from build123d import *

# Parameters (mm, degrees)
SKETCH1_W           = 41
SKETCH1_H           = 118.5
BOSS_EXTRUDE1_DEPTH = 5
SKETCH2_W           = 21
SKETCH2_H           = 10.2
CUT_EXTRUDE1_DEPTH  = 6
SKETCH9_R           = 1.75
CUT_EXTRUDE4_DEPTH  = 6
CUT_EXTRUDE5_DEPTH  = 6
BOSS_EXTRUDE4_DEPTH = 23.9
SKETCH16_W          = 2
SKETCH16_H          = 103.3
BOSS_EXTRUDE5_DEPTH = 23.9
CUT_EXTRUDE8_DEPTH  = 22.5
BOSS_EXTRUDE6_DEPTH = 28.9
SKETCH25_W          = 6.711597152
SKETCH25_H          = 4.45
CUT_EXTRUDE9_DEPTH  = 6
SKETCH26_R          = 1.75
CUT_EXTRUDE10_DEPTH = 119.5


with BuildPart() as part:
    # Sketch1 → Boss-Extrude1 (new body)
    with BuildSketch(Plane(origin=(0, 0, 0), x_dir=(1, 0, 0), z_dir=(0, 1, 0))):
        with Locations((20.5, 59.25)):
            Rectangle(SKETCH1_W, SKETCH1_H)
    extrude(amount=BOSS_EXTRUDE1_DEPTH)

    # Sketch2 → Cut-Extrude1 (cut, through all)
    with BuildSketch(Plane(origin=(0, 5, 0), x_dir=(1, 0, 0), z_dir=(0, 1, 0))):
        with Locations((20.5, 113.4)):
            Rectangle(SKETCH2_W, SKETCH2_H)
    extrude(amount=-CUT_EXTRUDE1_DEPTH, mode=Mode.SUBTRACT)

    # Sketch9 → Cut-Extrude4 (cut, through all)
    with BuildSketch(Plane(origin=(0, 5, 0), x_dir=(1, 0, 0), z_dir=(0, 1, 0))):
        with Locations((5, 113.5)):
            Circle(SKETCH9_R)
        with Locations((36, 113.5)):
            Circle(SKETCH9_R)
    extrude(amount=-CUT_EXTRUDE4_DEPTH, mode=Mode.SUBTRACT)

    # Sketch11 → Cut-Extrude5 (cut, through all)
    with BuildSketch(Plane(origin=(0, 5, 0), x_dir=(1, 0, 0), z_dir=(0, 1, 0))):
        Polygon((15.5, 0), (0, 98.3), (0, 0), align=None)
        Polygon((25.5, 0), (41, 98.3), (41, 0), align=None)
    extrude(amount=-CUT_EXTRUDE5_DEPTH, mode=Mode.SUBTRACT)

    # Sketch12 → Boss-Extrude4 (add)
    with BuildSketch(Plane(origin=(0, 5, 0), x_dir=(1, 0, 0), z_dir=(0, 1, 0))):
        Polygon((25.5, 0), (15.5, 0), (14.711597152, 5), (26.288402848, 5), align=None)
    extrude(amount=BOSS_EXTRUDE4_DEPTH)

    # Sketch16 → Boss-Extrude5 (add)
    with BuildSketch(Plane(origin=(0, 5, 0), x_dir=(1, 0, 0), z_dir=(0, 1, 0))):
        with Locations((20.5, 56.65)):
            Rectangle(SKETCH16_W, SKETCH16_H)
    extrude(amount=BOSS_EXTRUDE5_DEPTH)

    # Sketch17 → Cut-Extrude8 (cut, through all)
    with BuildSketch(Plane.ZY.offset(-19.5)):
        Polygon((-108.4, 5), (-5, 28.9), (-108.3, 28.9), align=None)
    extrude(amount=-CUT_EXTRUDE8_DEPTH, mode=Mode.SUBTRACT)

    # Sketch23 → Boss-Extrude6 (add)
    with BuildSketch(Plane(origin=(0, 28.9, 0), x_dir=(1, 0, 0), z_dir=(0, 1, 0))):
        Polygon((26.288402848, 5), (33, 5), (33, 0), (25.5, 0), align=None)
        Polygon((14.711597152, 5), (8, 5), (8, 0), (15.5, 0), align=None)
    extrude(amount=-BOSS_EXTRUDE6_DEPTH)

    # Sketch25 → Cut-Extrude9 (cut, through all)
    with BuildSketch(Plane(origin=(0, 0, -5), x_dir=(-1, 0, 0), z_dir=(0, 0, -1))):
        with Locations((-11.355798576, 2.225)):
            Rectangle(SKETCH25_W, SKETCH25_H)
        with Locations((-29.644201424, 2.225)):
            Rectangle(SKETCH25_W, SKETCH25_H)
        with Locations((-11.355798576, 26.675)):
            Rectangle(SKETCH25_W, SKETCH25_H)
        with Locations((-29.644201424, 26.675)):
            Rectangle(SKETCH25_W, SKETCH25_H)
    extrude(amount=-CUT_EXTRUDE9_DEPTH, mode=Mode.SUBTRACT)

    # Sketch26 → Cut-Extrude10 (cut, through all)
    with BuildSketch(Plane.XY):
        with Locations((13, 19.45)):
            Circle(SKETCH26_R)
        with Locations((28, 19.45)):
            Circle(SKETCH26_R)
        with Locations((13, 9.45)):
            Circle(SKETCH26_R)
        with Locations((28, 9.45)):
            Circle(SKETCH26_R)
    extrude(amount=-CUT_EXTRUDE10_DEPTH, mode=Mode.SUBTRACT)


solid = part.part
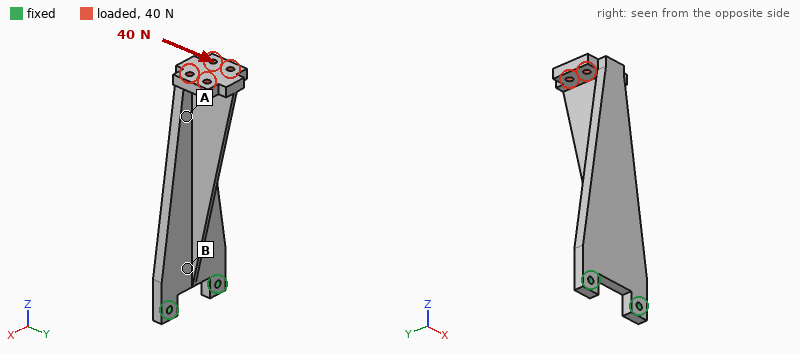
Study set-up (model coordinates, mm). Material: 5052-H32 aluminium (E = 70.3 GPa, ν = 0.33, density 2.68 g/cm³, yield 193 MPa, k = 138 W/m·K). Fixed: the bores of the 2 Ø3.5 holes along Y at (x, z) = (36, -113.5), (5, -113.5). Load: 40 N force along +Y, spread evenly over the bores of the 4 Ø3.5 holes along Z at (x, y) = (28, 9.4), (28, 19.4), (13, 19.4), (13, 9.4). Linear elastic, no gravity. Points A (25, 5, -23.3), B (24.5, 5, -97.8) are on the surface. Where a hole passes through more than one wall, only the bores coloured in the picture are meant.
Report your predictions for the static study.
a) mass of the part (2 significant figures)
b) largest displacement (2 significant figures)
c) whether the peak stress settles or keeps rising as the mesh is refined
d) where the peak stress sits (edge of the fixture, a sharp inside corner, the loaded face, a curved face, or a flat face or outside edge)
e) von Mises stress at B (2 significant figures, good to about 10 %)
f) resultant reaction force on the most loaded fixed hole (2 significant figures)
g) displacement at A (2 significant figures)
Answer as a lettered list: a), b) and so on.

a) 55 g
b) 0.60 mm
c) keeps rising
d) edge of the fixture
e) 15 MPa
f) 23 N
g) 0.44 mm
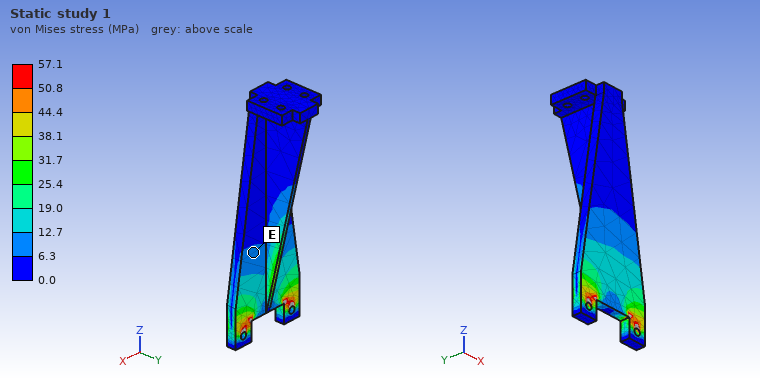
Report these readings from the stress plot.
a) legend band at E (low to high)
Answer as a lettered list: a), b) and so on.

a) 6.3 to 12.7 MPa
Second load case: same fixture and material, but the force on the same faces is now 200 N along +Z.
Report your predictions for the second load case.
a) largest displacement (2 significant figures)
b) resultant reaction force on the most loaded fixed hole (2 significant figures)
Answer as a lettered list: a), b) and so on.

a) 0.38 mm
b) 100 N
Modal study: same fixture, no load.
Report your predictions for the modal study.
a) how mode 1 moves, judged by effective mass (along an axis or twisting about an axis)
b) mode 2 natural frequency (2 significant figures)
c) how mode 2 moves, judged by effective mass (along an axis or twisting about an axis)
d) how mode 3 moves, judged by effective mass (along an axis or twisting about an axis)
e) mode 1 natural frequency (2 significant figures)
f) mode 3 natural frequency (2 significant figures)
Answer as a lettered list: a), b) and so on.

a) along Y
b) 1300 Hz
c) along X
d) along Y
e) 310 Hz
f) 2800 Hz
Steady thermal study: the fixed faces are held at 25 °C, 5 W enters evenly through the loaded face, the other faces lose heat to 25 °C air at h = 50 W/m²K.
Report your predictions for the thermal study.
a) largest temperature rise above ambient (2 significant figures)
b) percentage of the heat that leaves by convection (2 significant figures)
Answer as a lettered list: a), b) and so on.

a) 15 K
b) 69 %
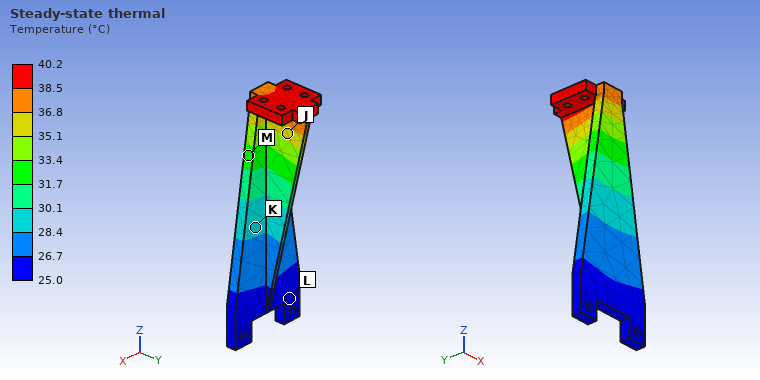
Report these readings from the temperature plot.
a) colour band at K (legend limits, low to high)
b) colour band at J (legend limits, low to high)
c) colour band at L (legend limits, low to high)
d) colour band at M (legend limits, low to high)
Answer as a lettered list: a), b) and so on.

a) 28.4 to 30.1 °C
b) 35.1 to 36.8 °C
c) 25.0 to 26.7 °C
d) 31.7 to 33.4 °C
